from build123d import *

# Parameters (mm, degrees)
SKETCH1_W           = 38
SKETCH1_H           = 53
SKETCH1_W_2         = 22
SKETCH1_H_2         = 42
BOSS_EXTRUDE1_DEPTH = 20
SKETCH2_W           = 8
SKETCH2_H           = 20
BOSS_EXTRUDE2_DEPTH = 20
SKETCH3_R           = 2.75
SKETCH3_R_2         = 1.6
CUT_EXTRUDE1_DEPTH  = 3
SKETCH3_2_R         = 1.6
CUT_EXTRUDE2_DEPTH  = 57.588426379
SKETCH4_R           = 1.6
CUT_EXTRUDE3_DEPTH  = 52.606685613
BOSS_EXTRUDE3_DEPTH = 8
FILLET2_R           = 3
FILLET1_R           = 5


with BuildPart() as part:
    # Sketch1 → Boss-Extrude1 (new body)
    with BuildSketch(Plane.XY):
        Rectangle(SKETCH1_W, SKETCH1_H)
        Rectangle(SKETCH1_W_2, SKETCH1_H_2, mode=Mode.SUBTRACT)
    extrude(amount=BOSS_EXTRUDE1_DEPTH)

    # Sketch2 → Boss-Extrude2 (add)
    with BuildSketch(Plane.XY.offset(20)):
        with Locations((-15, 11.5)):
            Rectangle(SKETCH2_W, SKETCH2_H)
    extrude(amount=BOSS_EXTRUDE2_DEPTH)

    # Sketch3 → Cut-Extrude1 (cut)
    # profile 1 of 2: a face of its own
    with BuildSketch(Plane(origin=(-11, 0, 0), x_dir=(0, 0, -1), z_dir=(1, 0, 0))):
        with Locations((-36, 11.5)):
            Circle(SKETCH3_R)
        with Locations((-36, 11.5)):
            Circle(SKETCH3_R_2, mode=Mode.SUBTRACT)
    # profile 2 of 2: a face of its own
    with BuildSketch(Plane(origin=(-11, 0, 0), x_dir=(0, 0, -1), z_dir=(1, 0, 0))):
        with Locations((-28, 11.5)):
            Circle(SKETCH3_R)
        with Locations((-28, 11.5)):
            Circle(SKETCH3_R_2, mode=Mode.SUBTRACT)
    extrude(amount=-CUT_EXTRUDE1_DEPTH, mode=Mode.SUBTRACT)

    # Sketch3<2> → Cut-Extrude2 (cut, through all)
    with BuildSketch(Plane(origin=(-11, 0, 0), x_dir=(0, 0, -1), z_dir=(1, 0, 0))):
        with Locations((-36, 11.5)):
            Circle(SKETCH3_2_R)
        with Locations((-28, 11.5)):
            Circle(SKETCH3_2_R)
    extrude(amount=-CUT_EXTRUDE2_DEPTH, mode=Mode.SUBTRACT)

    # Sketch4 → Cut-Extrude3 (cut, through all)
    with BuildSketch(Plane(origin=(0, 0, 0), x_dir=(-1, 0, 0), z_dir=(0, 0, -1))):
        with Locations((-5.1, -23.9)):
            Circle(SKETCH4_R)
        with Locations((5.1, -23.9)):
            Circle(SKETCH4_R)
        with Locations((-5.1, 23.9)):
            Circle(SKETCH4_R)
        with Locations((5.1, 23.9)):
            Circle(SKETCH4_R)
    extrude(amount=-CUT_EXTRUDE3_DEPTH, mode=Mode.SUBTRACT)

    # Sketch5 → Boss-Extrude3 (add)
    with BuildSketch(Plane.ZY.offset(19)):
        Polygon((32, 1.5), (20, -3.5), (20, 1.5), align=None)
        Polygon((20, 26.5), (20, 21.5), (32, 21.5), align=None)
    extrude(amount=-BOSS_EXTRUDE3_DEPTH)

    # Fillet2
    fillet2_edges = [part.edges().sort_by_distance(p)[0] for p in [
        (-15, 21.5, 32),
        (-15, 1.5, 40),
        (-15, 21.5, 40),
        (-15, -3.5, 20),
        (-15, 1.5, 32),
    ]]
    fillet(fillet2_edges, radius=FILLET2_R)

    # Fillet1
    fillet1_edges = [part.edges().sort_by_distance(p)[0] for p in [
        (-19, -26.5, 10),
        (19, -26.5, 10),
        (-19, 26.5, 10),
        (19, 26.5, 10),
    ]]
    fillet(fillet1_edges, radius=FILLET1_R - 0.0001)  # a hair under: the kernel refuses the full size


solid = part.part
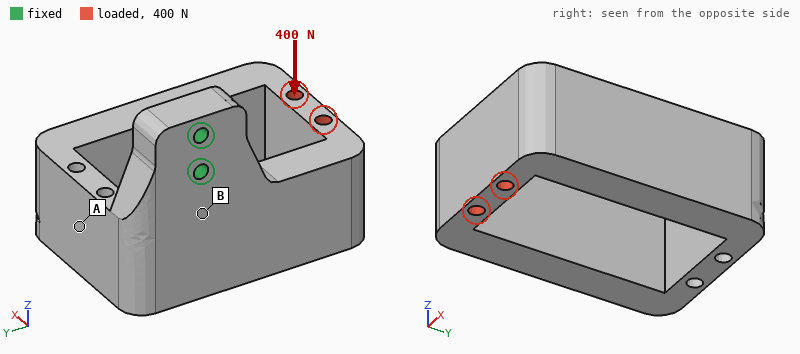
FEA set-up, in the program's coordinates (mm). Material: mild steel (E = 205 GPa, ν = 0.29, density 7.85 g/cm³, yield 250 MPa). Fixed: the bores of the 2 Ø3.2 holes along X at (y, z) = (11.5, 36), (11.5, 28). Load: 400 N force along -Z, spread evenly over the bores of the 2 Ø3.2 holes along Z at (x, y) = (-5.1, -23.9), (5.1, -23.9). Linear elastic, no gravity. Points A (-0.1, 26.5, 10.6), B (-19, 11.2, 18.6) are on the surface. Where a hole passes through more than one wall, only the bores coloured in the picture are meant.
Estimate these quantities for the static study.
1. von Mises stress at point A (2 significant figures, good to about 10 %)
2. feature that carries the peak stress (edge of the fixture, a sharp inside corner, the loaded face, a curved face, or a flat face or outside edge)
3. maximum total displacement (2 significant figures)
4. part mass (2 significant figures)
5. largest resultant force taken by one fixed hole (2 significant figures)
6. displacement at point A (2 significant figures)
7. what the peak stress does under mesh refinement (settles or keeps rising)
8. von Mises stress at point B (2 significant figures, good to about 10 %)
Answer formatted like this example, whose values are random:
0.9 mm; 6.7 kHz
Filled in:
7.1 MPa; edge of the fixture; 50 µm; 190 g; 1.4 kN; 9.3 µm; keeps rising; 18 MPa
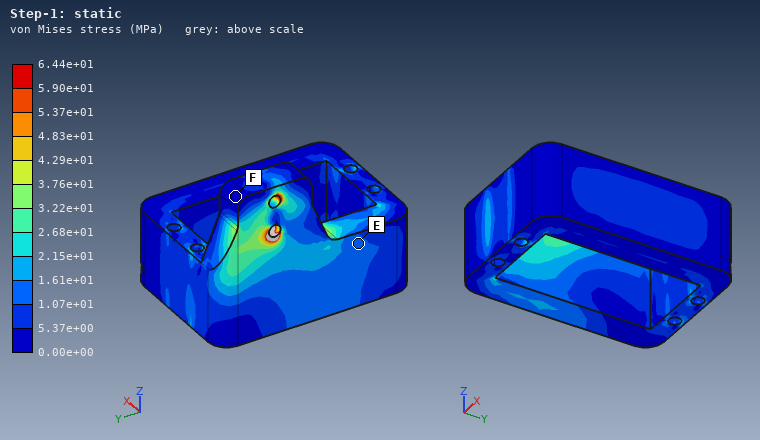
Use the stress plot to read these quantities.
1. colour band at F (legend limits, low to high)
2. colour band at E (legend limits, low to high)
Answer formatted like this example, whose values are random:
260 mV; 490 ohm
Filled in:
0.00e+00 to 5.37e+00 MPa; 1.07e+01 to 1.61e+01 MPa
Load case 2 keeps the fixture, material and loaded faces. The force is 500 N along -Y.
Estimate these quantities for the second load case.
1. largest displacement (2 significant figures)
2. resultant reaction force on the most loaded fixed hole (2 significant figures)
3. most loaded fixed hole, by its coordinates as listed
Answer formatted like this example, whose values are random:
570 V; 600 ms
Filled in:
50 µm; 1.2 kN; (11.5, 28)
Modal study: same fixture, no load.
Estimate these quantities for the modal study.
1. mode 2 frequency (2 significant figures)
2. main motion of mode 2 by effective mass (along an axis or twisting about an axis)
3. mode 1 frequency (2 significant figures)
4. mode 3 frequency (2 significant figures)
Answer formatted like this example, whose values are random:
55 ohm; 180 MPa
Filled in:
1500 Hz; along Z; 1200 Hz; 3300 Hz
